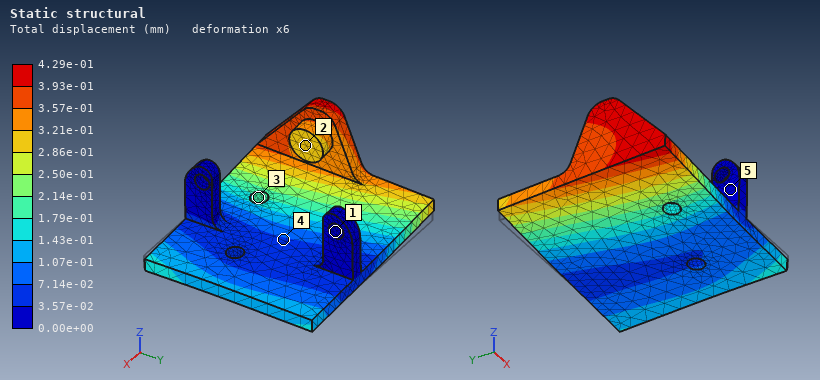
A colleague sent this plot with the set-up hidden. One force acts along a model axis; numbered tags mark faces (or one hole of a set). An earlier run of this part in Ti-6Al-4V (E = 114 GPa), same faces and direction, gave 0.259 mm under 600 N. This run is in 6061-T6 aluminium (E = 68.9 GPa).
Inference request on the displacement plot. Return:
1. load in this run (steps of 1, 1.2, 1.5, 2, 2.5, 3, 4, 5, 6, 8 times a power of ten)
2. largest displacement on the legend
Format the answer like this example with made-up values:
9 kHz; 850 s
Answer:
600 N; 4.29e-01 mm
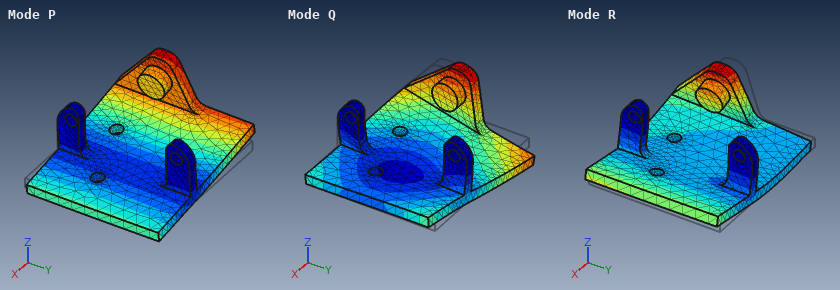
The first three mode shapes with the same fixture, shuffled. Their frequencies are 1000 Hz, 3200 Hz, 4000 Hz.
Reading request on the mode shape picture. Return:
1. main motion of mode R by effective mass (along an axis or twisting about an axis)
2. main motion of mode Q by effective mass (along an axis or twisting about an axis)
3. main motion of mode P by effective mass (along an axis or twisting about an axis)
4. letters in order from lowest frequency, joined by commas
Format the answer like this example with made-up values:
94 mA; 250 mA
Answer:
along X; along Y; along Z; P, Q, R
